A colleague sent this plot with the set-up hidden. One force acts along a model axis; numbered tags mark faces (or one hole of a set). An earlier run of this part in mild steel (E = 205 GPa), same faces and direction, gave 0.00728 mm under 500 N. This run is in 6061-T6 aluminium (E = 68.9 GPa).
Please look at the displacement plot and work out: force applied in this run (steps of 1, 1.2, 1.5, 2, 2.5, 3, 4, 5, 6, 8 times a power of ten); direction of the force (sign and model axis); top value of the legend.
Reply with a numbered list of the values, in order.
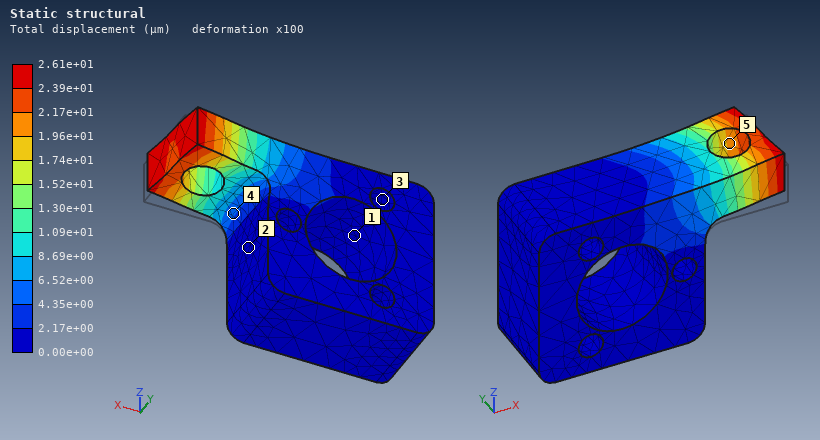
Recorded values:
1. 600 N
2. +Y
3. 2.61e+01 µm
